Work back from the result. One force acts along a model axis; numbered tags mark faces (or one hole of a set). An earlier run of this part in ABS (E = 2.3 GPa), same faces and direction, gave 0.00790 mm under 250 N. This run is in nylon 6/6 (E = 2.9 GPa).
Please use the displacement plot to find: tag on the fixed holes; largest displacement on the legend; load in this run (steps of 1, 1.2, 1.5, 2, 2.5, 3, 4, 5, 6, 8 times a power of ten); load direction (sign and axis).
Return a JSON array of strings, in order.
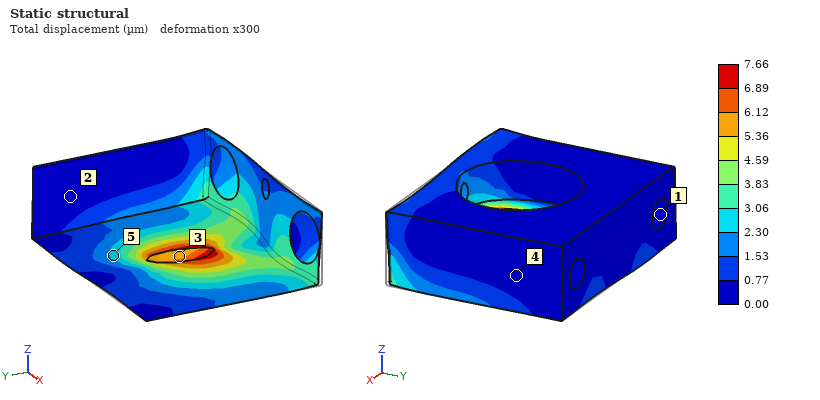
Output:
["1", "7.66 µm", "300 N", "-X"]
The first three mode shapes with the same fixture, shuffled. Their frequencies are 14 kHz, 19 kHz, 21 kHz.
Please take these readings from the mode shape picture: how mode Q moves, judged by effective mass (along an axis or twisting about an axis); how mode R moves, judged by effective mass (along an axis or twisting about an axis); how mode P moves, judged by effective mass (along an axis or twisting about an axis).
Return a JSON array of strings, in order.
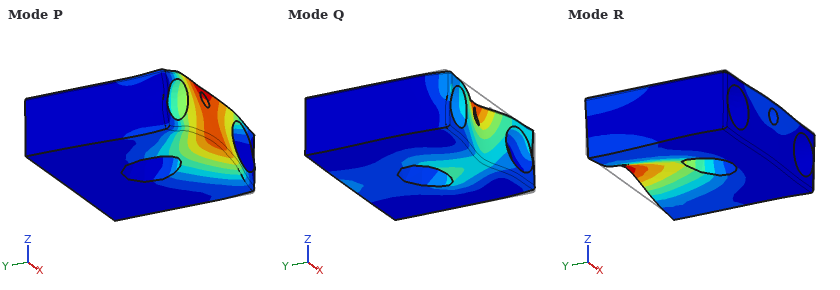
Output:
["along Y", "along Z", "along Z"]
